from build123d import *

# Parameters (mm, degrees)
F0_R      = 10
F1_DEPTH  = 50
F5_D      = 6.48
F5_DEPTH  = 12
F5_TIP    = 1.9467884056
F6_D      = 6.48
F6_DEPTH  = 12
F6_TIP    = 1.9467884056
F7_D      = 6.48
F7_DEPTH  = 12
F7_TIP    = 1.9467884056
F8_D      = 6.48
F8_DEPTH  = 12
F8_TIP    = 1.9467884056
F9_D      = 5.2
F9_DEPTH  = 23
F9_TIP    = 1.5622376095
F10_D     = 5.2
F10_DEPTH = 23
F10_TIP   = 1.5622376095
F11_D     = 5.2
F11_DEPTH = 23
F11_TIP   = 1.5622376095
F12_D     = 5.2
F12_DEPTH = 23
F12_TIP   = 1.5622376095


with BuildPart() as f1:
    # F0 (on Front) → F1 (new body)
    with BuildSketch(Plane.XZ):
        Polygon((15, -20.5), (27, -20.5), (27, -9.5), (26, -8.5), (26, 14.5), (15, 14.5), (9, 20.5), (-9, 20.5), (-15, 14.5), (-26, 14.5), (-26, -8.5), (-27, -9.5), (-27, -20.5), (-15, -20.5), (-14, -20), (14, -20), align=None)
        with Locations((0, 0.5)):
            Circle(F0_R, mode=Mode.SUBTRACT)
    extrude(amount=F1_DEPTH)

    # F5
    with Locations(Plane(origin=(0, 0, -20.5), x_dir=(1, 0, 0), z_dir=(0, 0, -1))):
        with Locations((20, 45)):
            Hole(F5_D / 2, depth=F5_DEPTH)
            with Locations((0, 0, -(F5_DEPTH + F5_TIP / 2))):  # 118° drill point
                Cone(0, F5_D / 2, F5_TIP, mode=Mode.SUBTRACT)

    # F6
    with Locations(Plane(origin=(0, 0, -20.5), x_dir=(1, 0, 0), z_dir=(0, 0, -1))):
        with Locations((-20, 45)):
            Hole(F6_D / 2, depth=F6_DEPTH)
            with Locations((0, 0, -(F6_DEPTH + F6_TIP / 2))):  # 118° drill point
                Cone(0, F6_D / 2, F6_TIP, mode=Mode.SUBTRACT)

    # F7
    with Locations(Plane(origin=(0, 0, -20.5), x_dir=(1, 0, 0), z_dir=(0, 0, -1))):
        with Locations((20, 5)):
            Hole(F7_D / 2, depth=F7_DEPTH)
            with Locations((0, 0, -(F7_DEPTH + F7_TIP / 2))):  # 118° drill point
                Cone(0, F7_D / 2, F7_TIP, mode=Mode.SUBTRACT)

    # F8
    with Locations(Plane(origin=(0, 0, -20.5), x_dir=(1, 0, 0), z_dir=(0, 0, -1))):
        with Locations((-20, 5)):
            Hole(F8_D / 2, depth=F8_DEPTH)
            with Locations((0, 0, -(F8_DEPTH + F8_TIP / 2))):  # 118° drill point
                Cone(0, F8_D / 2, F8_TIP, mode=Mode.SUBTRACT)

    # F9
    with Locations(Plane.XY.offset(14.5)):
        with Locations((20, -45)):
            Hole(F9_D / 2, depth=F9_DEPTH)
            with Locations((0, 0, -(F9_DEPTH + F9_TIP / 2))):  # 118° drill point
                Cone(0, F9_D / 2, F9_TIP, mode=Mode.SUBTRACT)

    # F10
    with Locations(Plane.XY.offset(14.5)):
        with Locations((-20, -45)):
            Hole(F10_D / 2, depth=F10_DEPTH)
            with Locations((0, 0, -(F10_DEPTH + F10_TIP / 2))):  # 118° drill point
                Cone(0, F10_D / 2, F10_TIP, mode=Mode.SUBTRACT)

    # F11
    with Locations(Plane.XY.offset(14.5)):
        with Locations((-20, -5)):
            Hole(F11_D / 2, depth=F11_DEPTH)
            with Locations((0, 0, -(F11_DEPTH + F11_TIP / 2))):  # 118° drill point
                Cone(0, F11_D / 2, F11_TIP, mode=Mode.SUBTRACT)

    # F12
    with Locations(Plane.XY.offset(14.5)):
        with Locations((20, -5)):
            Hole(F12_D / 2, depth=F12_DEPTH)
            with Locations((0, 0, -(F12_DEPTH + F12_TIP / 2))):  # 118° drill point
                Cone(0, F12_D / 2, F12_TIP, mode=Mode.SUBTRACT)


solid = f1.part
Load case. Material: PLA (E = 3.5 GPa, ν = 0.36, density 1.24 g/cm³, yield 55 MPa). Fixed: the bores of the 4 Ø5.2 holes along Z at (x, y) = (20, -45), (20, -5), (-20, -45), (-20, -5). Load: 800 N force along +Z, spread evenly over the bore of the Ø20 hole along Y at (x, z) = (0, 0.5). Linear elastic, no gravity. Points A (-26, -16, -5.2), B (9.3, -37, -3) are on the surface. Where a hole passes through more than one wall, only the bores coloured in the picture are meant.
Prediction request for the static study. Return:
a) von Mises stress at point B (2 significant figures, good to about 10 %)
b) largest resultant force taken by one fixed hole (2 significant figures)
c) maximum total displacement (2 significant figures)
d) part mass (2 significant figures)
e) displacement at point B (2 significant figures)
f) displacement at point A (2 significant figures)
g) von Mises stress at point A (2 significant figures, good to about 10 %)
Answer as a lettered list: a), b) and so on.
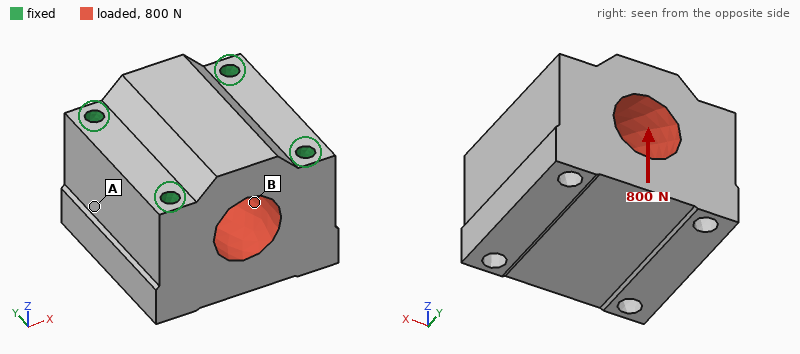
a) 0.56 MPa
b) 200 N
c) 5.8 µm
d) 98 g
e) 4.0 µm
f) 1.9 µm
g) 0.21 MPa
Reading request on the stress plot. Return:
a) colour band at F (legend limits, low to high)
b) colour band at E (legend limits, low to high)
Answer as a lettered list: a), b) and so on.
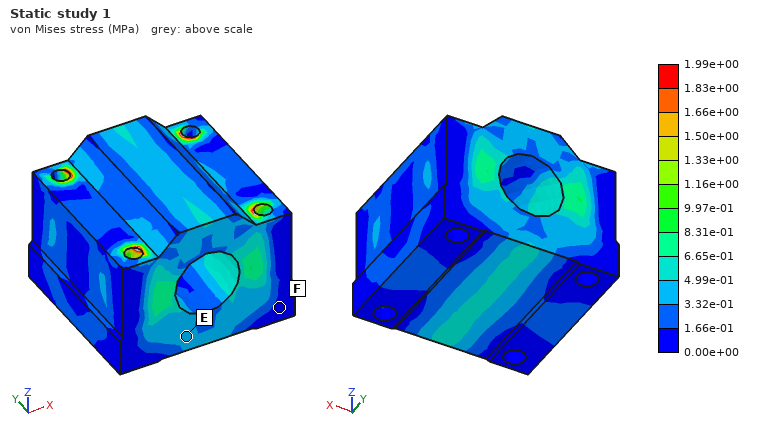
a) 0.00e+00 to 1.66e-01 MPa
b) 3.32e-01 to 4.99e-01 MPa
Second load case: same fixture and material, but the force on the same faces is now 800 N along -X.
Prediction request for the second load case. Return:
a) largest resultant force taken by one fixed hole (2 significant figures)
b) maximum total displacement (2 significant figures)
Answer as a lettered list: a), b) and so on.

a) 210 N
b) 4.0 µm
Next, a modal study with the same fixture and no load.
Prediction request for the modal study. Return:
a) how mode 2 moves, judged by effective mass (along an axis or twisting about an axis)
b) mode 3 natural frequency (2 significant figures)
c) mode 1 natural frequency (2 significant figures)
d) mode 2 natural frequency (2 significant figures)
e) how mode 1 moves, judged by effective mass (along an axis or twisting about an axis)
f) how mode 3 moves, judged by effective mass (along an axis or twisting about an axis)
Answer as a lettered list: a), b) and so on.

a) along Z
b) 8900 Hz
c) 7600 Hz
d) 8400 Hz
e) along X
f) along Y
